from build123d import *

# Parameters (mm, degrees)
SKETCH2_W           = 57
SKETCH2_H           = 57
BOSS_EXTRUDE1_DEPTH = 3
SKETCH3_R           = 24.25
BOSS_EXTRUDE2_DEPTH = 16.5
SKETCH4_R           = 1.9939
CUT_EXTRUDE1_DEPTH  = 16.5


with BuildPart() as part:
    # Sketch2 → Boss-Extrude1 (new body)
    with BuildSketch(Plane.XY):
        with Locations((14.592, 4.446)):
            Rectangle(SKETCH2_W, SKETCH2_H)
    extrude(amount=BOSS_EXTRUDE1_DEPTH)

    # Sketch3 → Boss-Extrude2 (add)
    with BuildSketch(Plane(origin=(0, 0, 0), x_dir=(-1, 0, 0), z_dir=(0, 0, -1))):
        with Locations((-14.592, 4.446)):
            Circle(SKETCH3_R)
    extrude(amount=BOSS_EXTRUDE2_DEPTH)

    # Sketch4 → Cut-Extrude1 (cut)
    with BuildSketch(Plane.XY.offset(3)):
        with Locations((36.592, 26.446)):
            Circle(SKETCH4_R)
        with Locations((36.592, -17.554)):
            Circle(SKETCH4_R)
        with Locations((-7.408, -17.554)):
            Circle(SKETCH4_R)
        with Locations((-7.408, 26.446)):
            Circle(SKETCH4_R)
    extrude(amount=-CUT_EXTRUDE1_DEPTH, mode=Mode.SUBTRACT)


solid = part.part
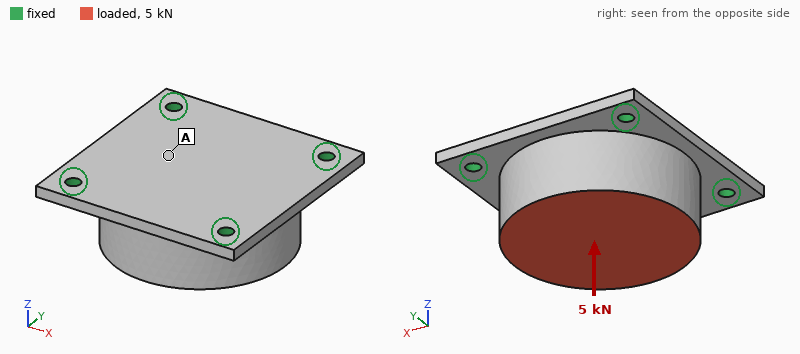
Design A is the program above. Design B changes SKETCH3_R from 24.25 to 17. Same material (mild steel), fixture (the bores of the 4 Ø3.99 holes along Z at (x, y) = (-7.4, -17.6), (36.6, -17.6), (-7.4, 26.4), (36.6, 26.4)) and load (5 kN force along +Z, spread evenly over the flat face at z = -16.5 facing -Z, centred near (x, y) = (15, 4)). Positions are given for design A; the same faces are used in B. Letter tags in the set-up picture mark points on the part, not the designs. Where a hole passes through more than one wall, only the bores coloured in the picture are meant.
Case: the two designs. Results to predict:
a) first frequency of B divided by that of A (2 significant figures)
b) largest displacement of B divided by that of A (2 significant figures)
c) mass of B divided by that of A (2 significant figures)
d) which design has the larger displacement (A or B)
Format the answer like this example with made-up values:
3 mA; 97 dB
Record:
0.68; 4.0; 0.61; B
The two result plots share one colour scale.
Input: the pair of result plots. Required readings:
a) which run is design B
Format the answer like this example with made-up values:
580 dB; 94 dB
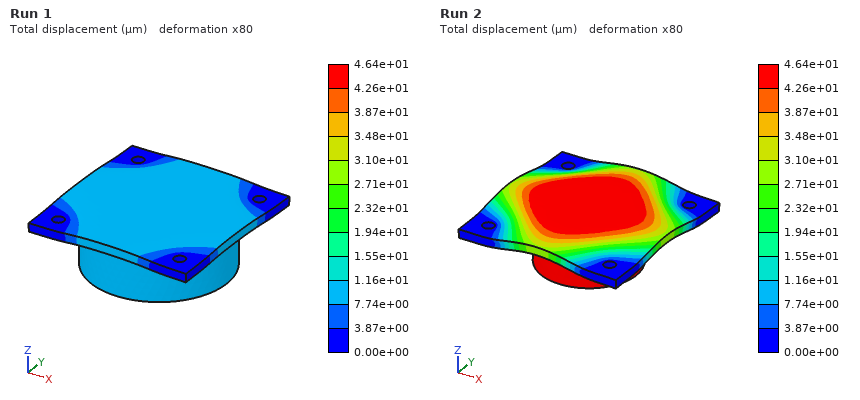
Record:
Run 2
